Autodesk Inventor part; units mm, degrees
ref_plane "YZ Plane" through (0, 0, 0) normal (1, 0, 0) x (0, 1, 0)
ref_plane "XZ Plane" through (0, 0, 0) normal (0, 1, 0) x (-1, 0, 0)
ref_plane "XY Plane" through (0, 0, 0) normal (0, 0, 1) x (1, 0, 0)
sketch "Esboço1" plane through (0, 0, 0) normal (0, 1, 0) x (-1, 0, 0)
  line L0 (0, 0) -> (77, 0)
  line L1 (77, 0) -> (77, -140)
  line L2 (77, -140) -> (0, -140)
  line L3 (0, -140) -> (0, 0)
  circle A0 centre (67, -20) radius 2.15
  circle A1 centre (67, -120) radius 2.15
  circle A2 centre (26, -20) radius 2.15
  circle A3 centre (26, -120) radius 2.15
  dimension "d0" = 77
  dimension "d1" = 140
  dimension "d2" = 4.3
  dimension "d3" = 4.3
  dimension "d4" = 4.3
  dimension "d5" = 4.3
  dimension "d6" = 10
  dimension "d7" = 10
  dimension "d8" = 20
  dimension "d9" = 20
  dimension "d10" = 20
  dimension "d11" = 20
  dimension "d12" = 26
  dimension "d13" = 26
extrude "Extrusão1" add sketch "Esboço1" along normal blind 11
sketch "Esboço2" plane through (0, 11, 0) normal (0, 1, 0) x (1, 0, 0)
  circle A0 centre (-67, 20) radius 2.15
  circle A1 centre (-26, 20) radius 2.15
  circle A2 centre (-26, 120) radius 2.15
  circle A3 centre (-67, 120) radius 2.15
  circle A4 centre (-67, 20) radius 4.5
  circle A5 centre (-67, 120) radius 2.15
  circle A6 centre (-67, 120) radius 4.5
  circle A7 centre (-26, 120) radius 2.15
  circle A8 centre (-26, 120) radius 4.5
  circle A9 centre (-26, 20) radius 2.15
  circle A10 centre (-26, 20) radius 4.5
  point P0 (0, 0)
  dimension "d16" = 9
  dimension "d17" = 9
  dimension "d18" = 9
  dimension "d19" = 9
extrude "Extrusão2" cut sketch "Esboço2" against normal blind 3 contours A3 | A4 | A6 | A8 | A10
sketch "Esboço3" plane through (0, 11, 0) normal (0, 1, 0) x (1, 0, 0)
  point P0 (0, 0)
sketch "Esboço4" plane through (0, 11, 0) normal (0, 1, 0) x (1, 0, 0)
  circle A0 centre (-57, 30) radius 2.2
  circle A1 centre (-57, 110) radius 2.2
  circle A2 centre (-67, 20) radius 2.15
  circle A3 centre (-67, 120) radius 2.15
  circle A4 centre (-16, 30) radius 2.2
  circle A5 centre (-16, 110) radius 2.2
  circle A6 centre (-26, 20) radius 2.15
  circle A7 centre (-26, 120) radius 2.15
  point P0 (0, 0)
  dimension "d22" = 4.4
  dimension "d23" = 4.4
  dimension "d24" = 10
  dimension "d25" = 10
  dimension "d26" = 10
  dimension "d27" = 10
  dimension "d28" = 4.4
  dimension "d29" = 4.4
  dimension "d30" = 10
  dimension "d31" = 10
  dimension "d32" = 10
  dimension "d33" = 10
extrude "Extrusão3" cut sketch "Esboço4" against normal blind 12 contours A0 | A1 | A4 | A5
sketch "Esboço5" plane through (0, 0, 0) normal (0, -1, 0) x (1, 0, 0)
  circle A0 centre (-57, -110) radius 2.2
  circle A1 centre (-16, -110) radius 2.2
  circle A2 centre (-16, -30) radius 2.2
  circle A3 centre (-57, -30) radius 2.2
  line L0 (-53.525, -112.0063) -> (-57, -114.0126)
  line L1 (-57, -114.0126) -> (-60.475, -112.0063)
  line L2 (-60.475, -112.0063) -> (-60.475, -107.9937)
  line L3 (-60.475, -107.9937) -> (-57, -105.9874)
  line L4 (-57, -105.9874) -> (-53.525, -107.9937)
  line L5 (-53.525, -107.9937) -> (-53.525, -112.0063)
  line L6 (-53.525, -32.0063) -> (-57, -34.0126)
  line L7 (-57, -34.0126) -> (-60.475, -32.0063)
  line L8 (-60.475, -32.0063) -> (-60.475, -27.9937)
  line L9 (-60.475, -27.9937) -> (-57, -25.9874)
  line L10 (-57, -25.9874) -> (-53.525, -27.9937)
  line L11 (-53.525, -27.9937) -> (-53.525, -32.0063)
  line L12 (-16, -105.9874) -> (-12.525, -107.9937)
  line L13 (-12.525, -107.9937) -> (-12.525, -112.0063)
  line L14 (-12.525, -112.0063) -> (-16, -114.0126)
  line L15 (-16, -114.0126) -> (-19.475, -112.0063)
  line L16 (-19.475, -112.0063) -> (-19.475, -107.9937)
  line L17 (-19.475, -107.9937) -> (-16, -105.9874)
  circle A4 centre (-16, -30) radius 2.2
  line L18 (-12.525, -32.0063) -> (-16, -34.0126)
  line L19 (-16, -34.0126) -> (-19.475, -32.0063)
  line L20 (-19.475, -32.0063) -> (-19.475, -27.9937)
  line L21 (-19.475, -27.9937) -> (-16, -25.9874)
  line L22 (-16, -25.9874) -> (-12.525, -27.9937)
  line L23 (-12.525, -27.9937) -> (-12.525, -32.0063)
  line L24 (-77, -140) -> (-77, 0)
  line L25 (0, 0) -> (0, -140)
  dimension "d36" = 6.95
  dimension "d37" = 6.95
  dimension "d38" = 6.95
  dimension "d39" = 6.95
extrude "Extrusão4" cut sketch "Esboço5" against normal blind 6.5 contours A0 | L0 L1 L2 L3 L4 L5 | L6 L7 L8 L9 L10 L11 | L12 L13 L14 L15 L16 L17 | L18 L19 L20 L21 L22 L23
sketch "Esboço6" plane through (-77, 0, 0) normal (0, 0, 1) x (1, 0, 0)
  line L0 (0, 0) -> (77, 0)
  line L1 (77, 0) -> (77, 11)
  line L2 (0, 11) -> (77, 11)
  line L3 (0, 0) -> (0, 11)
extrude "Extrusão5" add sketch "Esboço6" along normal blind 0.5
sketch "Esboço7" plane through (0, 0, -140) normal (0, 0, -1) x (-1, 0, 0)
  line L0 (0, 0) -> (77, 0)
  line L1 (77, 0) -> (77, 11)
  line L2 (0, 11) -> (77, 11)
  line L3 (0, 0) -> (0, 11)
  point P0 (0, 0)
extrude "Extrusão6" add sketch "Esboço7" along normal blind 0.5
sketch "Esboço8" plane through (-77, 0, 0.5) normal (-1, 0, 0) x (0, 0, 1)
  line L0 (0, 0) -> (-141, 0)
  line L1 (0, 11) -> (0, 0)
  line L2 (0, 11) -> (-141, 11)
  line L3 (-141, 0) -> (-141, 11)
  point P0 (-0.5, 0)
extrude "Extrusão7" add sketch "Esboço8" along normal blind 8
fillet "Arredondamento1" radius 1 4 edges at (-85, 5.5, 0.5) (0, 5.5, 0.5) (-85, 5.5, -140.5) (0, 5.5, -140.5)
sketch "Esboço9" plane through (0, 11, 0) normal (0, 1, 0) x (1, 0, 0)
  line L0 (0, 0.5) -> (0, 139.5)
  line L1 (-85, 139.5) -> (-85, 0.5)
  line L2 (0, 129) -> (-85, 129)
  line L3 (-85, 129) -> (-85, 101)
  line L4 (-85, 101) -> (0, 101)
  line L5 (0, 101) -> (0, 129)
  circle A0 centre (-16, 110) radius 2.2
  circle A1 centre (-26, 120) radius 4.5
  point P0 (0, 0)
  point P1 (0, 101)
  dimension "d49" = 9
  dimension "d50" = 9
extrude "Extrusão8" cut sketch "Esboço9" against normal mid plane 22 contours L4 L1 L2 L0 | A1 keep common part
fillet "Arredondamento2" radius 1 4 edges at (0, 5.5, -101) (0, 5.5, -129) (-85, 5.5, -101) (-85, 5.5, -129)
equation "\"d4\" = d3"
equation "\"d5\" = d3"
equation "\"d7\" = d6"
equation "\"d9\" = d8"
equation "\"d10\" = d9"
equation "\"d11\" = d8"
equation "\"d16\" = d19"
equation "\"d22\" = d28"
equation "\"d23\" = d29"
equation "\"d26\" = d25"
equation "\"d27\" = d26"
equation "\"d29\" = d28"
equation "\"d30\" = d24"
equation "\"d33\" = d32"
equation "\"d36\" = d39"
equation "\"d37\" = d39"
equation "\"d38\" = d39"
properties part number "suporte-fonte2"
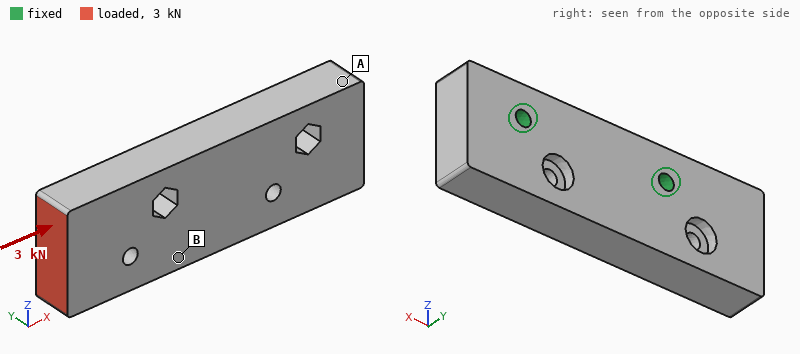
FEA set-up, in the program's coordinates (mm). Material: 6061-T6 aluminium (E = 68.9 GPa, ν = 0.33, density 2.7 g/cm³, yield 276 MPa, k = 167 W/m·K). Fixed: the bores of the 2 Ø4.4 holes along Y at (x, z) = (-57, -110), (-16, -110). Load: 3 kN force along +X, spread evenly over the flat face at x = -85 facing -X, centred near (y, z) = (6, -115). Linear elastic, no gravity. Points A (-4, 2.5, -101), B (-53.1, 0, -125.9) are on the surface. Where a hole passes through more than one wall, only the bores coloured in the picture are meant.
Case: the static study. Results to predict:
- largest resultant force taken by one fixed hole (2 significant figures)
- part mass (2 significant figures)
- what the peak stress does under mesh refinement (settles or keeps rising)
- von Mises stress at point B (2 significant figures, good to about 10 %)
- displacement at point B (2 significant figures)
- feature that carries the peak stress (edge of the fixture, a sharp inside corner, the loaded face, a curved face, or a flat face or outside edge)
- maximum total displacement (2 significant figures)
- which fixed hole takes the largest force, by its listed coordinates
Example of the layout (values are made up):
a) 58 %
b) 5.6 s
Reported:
a) 2.1 kN
b) 67 g
c) keeps rising
d) 14 MPa
e) 5.6 µm
f) edge of the fixture
g) 15 µm
h) (-57, -110)
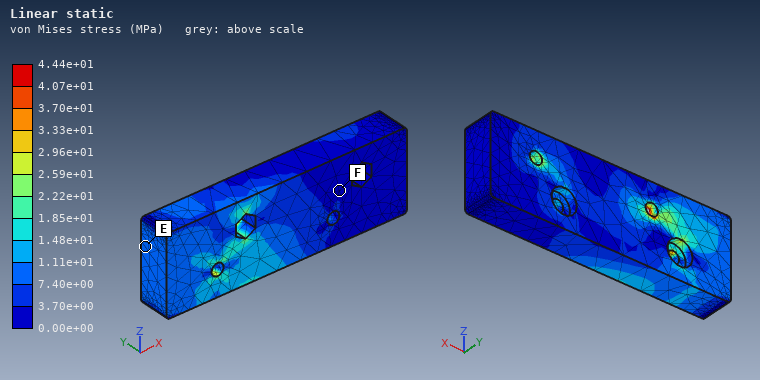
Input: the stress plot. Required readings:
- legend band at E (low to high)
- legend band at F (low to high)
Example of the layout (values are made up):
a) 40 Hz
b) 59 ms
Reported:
a) 7.40e+00 to 1.11e+01 MPa
b) 0.00e+00 to 3.70e+00 MPa
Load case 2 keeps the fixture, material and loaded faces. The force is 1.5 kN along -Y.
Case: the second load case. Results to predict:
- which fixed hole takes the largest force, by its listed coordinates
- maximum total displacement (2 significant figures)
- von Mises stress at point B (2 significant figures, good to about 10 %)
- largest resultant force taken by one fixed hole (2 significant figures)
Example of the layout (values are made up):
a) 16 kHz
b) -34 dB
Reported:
a) (-57, -110)
b) 0.14 mm
c) 49 MPa
d) 2.7 kN
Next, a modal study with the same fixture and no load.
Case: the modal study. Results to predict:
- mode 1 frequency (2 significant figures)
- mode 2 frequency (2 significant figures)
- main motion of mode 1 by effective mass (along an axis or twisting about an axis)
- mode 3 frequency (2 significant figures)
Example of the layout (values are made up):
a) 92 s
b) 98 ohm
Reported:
a) 5700 Hz
b) 6900 Hz
c) along Y
d) 10 kHz
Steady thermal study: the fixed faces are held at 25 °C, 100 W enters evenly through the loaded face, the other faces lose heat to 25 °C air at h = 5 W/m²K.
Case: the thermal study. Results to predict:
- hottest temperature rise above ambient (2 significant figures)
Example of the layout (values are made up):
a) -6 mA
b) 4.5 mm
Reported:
a) 77 K
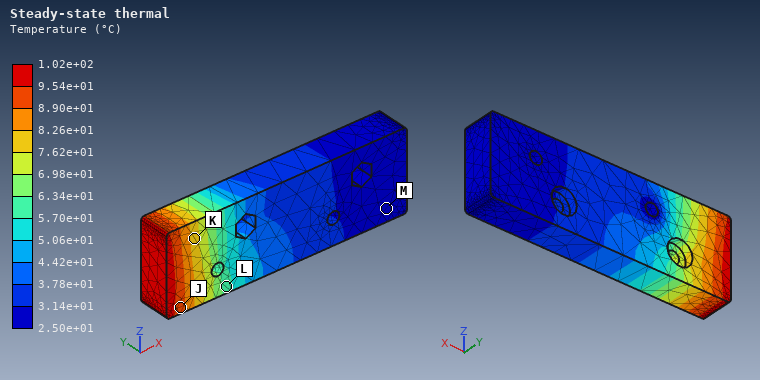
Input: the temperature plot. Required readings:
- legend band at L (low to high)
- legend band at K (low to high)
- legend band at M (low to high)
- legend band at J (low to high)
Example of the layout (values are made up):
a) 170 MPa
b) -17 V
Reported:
a) 5.70e+01 to 6.34e+01 °C
b) 7.62e+01 to 8.26e+01 °C
c) 2.50e+01 to 3.14e+01 °C
d) 8.90e+01 to 9.54e+01 °C
